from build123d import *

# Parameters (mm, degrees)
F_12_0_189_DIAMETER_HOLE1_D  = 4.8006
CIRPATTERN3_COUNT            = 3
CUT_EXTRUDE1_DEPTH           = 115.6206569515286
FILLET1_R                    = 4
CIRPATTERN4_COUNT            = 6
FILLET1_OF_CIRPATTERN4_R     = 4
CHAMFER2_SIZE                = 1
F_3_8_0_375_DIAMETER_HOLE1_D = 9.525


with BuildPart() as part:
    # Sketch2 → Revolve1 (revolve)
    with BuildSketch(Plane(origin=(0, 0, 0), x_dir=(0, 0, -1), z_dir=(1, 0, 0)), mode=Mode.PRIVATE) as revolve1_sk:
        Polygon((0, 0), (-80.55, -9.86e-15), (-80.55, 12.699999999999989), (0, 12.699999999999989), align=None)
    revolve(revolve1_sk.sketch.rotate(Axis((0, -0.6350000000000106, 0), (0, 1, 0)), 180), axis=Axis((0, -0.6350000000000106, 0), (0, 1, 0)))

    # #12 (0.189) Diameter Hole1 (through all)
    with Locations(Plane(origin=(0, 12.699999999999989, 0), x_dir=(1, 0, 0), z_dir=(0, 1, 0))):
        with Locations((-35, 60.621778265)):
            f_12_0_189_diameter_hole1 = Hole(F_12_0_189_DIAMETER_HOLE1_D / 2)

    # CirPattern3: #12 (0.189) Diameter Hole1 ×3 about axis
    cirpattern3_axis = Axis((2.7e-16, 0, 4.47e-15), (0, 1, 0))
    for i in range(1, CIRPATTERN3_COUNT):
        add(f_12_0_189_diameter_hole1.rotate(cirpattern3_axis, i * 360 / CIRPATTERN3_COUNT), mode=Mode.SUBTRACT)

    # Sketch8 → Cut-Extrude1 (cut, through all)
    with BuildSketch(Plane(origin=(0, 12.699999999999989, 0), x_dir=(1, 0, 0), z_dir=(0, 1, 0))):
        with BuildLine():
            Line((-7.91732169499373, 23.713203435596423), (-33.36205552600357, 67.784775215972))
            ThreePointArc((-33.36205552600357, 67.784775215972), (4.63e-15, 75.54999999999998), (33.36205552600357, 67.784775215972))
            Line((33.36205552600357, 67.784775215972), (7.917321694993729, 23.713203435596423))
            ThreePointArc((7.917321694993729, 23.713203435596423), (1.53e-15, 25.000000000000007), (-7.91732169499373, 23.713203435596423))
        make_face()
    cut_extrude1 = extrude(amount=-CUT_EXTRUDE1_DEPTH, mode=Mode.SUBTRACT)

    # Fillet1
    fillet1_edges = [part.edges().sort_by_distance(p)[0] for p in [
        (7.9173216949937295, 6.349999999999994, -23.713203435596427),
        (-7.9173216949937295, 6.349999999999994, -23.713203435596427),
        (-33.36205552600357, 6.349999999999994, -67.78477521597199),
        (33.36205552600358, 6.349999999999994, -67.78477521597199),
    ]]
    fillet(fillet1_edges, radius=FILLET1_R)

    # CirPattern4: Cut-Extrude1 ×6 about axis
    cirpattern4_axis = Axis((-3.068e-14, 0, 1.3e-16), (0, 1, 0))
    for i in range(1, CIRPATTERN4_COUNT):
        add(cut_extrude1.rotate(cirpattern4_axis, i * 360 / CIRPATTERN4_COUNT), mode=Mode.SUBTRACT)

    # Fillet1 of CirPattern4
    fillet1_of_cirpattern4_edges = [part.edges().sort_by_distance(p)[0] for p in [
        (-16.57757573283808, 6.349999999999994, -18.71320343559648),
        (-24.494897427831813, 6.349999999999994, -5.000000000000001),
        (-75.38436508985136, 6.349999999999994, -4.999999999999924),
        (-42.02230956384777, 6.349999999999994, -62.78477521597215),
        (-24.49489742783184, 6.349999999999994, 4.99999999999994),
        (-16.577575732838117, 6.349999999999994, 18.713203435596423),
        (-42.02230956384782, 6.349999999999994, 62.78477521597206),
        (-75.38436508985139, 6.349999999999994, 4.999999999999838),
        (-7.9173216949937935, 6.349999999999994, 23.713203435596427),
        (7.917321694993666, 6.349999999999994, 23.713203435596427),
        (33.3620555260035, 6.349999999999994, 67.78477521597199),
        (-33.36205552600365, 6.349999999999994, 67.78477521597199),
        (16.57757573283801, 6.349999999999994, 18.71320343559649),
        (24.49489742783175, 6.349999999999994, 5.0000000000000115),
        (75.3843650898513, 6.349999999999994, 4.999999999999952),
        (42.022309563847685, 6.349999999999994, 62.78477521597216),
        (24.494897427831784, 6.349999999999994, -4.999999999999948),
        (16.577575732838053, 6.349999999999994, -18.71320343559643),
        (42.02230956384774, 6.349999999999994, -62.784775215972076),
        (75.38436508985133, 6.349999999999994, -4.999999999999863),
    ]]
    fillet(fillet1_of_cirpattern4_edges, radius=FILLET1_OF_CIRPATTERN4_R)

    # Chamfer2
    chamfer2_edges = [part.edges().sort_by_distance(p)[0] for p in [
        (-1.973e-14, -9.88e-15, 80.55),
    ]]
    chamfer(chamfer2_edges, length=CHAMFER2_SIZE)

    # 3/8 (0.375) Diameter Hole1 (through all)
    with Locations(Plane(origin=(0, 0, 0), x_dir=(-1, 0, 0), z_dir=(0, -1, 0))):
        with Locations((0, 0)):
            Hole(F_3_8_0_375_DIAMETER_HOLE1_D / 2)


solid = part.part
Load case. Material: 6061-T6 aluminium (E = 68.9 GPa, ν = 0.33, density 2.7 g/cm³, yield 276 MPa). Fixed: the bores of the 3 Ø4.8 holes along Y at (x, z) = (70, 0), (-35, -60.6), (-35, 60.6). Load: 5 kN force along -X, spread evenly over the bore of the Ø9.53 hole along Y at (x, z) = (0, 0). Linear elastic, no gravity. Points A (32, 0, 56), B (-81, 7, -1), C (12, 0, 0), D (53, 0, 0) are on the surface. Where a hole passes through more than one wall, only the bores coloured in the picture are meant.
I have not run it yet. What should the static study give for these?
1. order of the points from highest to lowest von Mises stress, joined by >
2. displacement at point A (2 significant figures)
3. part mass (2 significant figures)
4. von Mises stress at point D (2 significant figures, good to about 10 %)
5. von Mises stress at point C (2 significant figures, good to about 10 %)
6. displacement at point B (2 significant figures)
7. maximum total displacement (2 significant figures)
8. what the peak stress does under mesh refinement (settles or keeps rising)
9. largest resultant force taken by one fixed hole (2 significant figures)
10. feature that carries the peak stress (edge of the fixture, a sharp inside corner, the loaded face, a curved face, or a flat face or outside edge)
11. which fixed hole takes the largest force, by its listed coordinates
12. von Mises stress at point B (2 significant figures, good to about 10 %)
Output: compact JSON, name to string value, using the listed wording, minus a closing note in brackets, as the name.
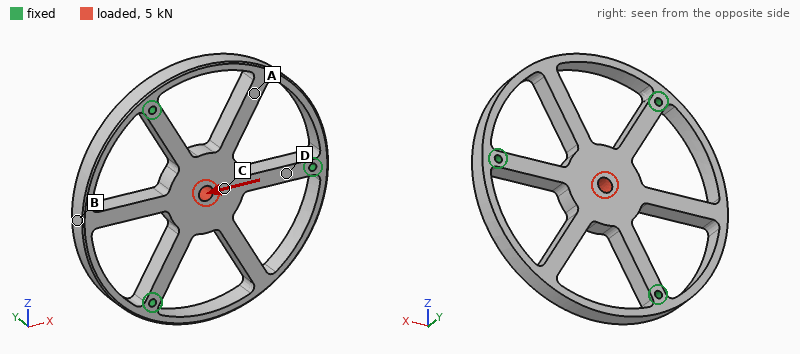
{"order of the points from highest to lowest von Mises stress, joined by >": "D > C > B > A", "displacement at point A": "13 µm", "part mass": "250 g", "von Mises stress at point D": "24 MPa", "von Mises stress at point C": "17 MPa", "displacement at point B": "20 µm", "maximum total displacement": "22 µm", "what the peak stress does under mesh refinement": "keeps rising", "largest resultant force taken by one fixed hole": "3.0 kN", "feature that carries the peak stress": "edge of the fixture", "which fixed hole takes the largest force, by its listed coordinates": "(70, 0)", "von Mises stress at point B": "8.1 MPa"}
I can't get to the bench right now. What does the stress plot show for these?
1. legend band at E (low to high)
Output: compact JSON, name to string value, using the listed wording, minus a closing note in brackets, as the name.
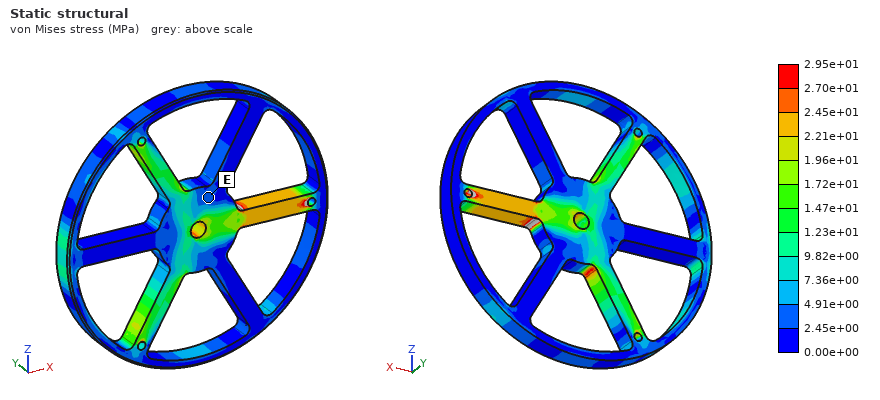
{"legend band at E": "2.45e+00 to 4.91e+00 MPa"}
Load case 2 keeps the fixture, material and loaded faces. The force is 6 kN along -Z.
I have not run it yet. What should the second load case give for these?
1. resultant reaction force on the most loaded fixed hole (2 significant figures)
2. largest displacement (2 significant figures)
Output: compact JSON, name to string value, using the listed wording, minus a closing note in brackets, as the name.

{"resultant reaction force on the most loaded fixed hole": "3.2 kN", "largest displacement": "27 µm"}
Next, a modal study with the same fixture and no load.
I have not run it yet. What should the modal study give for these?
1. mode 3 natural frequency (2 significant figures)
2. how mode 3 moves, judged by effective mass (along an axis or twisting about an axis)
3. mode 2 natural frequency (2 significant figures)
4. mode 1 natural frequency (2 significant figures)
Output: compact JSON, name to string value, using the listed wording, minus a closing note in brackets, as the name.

{"mode 3 natural frequency": "2000 Hz", "how mode 3 moves, judged by effective mass": "along Y", "mode 2 natural frequency": "1900 Hz", "mode 1 natural frequency": "1900 Hz"}
